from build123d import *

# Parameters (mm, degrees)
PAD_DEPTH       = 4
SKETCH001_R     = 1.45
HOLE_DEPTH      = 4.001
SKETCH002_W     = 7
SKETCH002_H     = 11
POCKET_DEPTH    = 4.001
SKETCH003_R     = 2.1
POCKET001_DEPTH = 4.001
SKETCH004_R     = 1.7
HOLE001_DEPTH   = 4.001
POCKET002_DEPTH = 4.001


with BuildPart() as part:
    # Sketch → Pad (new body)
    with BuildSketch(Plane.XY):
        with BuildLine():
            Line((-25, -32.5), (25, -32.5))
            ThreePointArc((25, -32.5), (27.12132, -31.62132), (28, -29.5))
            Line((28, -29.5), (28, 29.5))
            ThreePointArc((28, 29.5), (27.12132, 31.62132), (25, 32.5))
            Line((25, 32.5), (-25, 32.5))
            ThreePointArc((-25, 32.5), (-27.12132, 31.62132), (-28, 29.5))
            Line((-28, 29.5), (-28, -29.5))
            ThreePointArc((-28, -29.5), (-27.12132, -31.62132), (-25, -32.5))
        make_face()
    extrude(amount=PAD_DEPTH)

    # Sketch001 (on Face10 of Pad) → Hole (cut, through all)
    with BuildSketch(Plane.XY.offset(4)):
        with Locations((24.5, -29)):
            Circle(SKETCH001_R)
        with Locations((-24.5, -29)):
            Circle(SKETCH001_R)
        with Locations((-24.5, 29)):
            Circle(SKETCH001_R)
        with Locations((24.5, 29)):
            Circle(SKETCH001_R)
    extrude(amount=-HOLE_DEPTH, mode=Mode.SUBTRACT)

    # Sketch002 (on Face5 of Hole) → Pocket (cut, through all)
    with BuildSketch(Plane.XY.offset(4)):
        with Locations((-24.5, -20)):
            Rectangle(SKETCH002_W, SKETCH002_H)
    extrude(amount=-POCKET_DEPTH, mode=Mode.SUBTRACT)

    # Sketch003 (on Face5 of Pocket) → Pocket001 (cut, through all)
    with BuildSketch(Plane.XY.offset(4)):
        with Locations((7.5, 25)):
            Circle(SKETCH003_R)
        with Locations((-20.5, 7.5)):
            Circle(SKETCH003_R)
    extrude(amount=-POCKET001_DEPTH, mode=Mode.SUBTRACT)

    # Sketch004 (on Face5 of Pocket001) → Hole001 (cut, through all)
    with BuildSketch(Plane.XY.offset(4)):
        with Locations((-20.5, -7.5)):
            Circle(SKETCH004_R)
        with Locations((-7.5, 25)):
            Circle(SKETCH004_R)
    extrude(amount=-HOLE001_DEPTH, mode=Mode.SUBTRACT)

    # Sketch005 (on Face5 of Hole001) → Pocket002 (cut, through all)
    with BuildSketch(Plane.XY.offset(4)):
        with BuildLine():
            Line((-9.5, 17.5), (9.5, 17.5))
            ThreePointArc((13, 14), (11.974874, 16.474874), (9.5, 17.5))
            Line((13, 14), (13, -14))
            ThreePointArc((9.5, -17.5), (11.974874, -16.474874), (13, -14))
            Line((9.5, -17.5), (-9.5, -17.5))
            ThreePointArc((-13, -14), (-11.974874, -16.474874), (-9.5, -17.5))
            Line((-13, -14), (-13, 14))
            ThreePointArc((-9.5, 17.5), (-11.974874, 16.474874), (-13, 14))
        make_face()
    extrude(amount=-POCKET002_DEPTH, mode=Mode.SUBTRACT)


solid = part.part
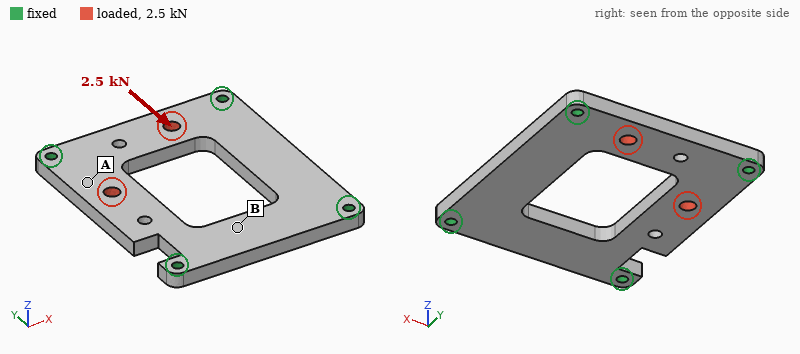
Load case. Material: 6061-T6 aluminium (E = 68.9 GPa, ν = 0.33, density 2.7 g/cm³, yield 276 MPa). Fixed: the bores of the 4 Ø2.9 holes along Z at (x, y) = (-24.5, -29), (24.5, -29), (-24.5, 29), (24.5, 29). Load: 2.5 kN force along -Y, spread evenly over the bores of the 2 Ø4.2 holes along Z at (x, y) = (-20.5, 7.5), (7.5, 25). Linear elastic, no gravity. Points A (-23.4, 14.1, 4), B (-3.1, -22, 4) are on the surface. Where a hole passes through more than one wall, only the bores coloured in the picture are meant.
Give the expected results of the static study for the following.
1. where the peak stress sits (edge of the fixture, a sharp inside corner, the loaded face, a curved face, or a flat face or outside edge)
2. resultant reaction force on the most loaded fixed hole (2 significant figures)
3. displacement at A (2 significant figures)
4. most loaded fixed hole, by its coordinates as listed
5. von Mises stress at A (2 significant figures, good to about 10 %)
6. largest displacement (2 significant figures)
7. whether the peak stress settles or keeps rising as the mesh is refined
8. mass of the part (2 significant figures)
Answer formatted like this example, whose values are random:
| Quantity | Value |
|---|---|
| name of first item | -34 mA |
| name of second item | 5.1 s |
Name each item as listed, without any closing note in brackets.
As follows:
| Quantity | Value |
|---|---|
| where the peak stress sits | edge of the fixture |
| resultant reaction force on the most loaded fixed hole | 1.2 kN |
| displacement at A | 8.7 µm |
| most loaded fixed hole, by its coordinates as listed | (-24.5, 29) |
| von Mises stress at A | 24 MPa |
| largest displacement | 21 µm |
| whether the peak stress settles or keeps rising as the mesh is refined | keeps rising |
| mass of the part | 28 g |
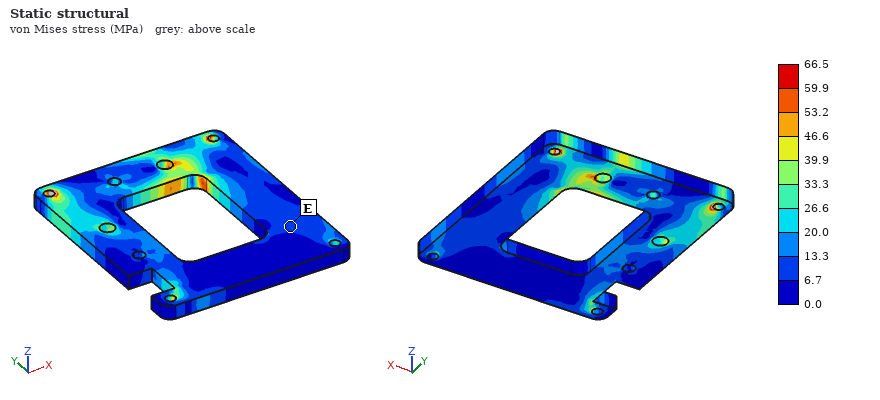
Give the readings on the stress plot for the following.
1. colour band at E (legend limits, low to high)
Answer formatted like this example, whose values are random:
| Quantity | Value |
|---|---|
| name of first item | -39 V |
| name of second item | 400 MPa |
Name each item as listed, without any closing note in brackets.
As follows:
| Quantity | Value |
|---|---|
| colour band at E | 6.7 to 13.3 MPa |
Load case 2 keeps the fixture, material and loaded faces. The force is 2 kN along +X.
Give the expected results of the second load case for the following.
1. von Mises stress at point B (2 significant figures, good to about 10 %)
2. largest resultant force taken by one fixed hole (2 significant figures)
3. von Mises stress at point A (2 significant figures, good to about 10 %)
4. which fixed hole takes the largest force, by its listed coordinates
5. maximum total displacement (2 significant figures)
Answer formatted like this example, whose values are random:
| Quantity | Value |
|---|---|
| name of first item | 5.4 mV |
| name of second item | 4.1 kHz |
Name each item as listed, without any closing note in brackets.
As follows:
| Quantity | Value |
|---|---|
| von Mises stress at point B | 8.3 MPa |
| largest resultant force taken by one fixed hole | 960 N |
| von Mises stress at point A | 22 MPa |
| which fixed hole takes the largest force, by its listed coordinates | (24.5, 29) |
| maximum total displacement | 22 µm |
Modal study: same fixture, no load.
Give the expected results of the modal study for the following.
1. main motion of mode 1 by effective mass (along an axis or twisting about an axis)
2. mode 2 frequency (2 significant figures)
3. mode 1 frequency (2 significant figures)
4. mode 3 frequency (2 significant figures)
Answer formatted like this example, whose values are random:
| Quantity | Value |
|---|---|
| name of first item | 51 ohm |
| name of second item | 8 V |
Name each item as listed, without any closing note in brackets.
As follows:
| Quantity | Value |
|---|---|
| main motion of mode 1 by effective mass | along Z |
| mode 2 frequency | 5900 Hz |
| mode 1 frequency | 4700 Hz |
| mode 3 frequency | 7700 Hz |
